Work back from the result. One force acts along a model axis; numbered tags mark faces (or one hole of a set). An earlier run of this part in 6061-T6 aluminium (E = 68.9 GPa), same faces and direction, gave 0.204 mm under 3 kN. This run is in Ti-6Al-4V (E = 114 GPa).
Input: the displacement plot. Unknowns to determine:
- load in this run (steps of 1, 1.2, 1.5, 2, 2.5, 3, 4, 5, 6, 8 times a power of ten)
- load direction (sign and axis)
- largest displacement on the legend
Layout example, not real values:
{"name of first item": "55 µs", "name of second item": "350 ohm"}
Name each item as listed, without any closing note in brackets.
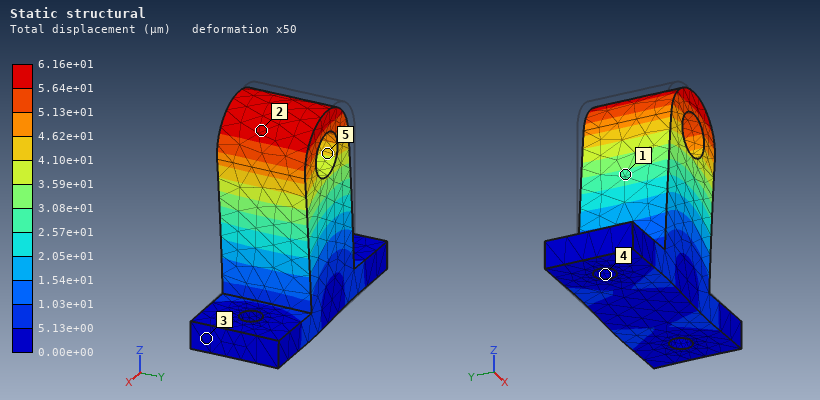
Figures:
{"load in this run": "1.5 kN", "load direction": "+X", "largest displacement on the legend": "6.16e+01 µm"}
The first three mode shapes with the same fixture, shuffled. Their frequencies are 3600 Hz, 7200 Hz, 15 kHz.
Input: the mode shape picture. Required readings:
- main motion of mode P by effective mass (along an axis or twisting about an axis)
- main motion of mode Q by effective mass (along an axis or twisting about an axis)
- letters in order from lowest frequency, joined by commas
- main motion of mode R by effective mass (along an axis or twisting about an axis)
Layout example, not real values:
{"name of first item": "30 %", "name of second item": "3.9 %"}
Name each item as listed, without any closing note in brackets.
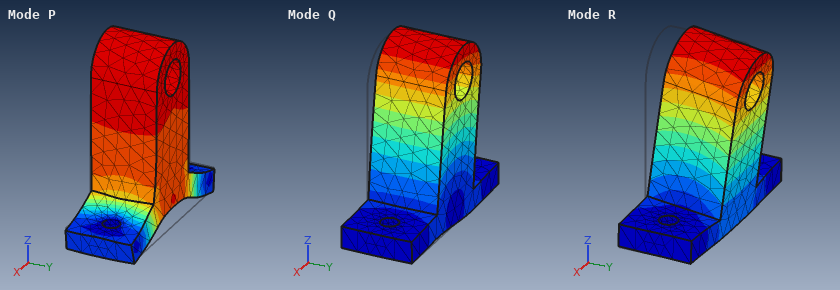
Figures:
{"main motion of mode P by effective mass": "along Z", "main motion of mode Q by effective mass": "along X", "letters in order from lowest frequency, joined by commas": "R, Q, P", "main motion of mode R by effective mass": "along Y"}
